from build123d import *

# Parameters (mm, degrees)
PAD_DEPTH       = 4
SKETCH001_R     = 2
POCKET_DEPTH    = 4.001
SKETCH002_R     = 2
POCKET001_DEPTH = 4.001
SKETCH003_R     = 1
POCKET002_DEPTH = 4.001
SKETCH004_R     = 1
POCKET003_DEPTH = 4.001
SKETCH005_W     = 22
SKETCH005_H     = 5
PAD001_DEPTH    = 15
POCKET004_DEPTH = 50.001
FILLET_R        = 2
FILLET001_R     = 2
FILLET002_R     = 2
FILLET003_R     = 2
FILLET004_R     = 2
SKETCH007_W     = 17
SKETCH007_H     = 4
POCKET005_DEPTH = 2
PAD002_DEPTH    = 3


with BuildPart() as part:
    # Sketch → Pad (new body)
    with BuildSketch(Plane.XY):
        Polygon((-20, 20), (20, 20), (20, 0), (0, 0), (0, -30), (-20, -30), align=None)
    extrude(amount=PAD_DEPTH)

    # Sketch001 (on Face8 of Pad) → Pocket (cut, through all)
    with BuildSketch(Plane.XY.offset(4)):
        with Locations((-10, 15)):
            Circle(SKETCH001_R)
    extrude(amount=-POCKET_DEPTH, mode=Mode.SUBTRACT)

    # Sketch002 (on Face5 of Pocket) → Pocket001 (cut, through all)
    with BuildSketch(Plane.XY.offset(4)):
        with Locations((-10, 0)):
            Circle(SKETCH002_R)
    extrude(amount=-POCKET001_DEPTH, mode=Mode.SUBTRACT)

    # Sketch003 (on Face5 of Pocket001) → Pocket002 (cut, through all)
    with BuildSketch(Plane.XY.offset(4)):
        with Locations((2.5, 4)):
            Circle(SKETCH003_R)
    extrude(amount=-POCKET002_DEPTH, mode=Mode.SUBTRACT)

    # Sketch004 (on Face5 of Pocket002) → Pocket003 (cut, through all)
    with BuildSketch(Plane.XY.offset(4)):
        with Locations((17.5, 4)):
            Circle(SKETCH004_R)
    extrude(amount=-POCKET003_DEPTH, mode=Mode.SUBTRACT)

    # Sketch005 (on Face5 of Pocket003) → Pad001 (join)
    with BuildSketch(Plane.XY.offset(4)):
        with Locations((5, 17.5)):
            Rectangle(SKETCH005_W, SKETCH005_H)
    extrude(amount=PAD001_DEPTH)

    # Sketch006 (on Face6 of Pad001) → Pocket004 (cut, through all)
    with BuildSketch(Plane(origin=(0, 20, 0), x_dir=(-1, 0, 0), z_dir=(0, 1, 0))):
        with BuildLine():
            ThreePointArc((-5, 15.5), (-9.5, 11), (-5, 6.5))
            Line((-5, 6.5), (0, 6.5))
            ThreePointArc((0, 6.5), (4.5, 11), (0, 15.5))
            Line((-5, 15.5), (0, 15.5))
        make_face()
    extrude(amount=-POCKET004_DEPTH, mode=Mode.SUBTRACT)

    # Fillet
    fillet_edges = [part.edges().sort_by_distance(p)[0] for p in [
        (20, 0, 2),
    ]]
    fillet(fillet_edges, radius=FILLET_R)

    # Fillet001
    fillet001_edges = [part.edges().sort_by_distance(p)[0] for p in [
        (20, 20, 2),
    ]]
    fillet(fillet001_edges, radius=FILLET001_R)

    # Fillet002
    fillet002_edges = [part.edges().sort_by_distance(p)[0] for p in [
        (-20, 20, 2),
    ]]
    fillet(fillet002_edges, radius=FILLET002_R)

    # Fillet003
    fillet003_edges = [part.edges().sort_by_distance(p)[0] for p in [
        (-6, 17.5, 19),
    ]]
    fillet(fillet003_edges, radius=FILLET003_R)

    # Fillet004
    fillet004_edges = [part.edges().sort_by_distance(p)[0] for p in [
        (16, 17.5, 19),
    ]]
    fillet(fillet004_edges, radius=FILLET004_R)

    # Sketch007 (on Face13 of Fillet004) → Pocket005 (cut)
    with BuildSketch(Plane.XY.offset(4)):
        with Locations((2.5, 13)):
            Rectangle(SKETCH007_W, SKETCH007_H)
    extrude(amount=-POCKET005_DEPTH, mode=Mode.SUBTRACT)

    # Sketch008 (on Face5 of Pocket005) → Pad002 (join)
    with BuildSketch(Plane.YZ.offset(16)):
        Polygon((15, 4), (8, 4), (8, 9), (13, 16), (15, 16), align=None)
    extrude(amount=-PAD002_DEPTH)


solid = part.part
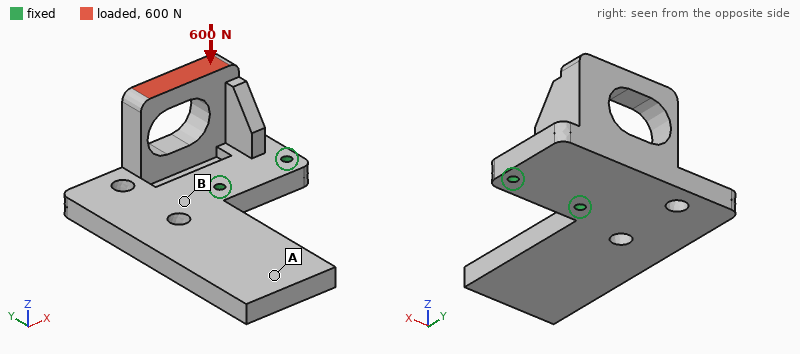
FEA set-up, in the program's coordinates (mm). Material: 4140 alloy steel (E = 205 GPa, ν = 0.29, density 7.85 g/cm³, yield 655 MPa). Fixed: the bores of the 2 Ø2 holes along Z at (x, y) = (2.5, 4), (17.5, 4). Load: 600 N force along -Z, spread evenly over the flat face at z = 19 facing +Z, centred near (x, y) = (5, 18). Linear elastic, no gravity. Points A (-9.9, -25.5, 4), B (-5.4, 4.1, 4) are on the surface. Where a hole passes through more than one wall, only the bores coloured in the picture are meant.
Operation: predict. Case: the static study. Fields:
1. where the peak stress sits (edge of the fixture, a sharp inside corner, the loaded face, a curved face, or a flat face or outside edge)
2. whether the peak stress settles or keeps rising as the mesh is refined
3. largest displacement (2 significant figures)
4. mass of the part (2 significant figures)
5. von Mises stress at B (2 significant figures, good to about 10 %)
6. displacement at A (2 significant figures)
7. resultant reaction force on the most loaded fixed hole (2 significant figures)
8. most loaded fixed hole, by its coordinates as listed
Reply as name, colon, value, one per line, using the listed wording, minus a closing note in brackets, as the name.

where the peak stress sits: edge of the fixture
whether the peak stress settles or keeps rising as the mesh is refined: keeps rising
largest displacement: 53 µm
mass of the part: 52 g
von Mises stress at B: 36 MPa
displacement at A: 37 µm
resultant reaction force on the most loaded fixed hole: 450 N
most loaded fixed hole, by its coordinates as listed: (2.5, 4)
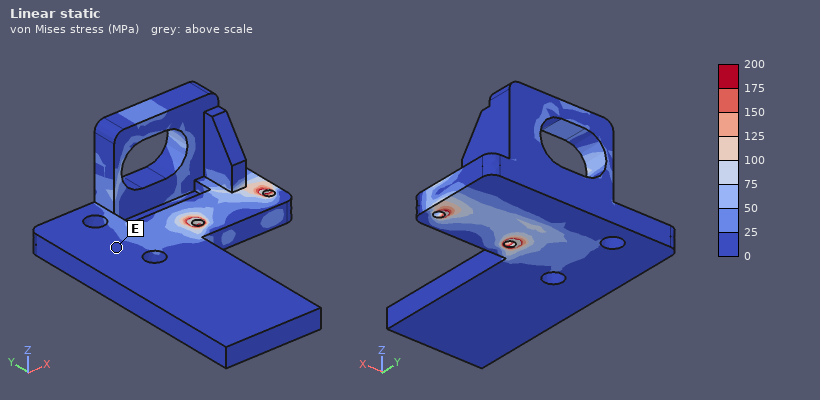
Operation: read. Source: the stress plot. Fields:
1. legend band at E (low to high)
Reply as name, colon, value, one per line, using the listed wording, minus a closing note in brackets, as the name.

legend band at E: 0 to 25 MPa
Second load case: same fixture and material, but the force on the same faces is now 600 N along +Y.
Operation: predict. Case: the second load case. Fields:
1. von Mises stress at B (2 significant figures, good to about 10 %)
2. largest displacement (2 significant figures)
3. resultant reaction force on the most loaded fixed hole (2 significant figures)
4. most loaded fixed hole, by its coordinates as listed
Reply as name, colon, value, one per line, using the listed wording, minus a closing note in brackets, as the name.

von Mises stress at B: 49 MPa
largest displacement: 0.12 mm
resultant reaction force on the most loaded fixed hole: 470 N
most loaded fixed hole, by its coordinates as listed: (2.5, 4)
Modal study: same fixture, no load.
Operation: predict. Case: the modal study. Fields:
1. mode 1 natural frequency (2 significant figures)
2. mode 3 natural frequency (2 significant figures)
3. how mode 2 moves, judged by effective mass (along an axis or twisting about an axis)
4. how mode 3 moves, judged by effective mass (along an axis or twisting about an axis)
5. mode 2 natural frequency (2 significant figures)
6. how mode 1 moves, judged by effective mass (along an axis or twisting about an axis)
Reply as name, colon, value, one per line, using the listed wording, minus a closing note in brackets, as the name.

mode 1 natural frequency: 1800 Hz
mode 3 natural frequency: 4900 Hz
how mode 2 moves, judged by effective mass: along Z
how mode 3 moves, judged by effective mass: along Y
mode 2 natural frequency: 4400 Hz
how mode 1 moves, judged by effective mass: along Z
